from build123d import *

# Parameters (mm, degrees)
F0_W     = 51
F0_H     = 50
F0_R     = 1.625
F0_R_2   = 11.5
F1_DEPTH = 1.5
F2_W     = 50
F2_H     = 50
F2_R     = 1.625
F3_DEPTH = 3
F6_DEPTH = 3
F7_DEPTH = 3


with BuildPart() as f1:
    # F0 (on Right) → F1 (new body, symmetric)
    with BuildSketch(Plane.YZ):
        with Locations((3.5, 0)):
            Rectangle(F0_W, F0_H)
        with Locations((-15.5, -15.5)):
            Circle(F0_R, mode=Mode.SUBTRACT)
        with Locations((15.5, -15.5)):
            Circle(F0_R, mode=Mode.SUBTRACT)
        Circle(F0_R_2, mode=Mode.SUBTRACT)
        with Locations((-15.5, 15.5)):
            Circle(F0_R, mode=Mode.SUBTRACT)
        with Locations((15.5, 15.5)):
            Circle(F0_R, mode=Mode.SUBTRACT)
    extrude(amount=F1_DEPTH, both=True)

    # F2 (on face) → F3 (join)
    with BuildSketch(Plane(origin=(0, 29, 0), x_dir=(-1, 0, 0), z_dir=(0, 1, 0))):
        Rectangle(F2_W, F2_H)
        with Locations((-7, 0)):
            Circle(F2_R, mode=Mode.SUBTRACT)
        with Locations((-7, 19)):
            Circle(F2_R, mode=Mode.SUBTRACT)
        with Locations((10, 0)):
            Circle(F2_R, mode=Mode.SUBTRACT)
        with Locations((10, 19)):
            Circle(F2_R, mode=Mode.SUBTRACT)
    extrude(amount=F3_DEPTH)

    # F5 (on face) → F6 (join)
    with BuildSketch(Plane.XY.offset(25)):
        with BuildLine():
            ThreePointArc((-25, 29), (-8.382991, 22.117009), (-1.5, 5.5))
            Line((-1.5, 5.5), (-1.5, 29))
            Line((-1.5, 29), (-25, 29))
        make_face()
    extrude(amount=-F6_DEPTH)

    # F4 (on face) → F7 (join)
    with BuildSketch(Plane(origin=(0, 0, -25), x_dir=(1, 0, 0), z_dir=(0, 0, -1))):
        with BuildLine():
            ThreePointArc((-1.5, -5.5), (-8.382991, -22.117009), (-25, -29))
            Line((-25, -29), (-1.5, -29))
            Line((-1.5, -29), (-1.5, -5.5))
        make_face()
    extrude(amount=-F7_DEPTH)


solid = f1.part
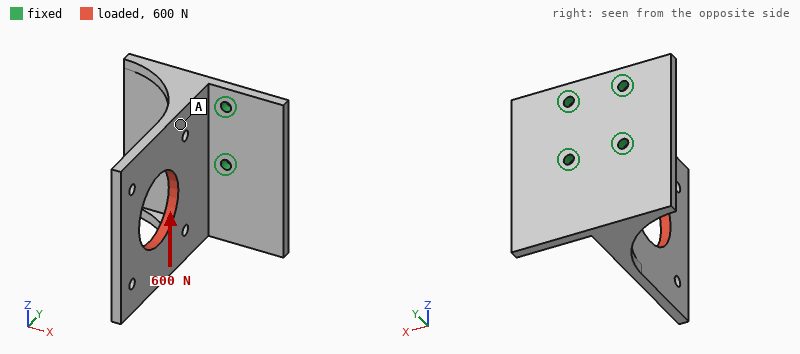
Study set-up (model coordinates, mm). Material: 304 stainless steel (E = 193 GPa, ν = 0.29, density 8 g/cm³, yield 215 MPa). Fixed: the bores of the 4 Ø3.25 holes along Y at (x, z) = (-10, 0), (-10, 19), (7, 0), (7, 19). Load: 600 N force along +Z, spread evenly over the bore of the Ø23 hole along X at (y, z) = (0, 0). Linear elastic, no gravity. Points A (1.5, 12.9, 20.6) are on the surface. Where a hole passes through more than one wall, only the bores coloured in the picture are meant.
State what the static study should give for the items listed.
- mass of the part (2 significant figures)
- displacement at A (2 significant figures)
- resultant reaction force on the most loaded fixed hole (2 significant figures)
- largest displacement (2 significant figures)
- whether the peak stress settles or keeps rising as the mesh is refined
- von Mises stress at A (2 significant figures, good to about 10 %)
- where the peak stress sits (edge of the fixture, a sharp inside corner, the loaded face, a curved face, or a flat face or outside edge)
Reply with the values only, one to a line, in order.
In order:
120 g
11 µm
530 N
34 µm
keeps rising
10 MPa
edge of the fixture
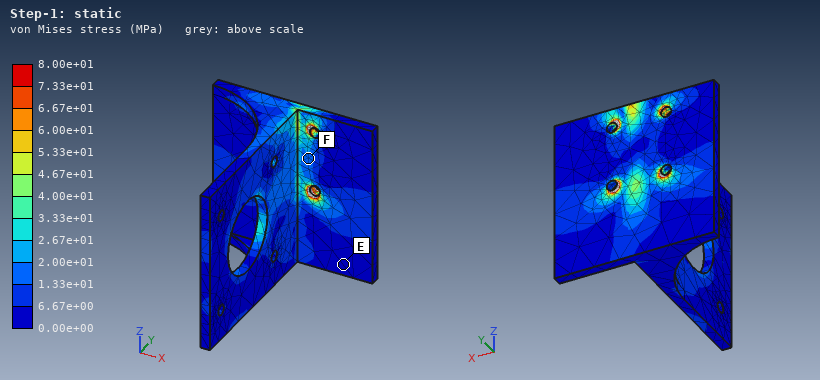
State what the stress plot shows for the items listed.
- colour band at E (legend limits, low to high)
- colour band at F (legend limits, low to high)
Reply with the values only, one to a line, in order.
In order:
0.00e+00 to 6.67e+00 MPa
1.33e+01 to 2.00e+01 MPa
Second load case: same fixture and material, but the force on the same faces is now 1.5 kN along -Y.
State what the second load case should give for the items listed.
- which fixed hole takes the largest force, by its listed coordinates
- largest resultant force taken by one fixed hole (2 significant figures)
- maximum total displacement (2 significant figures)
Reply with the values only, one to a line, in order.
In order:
(7, 0)
850 N
24 µm
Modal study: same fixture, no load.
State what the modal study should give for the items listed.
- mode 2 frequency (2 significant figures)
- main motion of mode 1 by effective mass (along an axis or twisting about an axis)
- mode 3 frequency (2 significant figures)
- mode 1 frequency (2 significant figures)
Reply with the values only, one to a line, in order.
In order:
2400 Hz
along X
3500 Hz
1100 Hz
